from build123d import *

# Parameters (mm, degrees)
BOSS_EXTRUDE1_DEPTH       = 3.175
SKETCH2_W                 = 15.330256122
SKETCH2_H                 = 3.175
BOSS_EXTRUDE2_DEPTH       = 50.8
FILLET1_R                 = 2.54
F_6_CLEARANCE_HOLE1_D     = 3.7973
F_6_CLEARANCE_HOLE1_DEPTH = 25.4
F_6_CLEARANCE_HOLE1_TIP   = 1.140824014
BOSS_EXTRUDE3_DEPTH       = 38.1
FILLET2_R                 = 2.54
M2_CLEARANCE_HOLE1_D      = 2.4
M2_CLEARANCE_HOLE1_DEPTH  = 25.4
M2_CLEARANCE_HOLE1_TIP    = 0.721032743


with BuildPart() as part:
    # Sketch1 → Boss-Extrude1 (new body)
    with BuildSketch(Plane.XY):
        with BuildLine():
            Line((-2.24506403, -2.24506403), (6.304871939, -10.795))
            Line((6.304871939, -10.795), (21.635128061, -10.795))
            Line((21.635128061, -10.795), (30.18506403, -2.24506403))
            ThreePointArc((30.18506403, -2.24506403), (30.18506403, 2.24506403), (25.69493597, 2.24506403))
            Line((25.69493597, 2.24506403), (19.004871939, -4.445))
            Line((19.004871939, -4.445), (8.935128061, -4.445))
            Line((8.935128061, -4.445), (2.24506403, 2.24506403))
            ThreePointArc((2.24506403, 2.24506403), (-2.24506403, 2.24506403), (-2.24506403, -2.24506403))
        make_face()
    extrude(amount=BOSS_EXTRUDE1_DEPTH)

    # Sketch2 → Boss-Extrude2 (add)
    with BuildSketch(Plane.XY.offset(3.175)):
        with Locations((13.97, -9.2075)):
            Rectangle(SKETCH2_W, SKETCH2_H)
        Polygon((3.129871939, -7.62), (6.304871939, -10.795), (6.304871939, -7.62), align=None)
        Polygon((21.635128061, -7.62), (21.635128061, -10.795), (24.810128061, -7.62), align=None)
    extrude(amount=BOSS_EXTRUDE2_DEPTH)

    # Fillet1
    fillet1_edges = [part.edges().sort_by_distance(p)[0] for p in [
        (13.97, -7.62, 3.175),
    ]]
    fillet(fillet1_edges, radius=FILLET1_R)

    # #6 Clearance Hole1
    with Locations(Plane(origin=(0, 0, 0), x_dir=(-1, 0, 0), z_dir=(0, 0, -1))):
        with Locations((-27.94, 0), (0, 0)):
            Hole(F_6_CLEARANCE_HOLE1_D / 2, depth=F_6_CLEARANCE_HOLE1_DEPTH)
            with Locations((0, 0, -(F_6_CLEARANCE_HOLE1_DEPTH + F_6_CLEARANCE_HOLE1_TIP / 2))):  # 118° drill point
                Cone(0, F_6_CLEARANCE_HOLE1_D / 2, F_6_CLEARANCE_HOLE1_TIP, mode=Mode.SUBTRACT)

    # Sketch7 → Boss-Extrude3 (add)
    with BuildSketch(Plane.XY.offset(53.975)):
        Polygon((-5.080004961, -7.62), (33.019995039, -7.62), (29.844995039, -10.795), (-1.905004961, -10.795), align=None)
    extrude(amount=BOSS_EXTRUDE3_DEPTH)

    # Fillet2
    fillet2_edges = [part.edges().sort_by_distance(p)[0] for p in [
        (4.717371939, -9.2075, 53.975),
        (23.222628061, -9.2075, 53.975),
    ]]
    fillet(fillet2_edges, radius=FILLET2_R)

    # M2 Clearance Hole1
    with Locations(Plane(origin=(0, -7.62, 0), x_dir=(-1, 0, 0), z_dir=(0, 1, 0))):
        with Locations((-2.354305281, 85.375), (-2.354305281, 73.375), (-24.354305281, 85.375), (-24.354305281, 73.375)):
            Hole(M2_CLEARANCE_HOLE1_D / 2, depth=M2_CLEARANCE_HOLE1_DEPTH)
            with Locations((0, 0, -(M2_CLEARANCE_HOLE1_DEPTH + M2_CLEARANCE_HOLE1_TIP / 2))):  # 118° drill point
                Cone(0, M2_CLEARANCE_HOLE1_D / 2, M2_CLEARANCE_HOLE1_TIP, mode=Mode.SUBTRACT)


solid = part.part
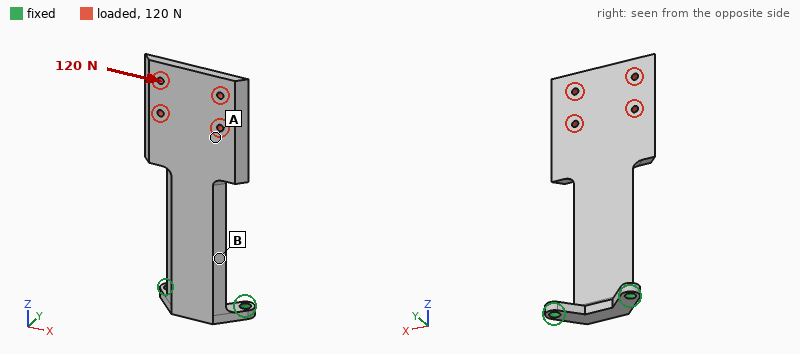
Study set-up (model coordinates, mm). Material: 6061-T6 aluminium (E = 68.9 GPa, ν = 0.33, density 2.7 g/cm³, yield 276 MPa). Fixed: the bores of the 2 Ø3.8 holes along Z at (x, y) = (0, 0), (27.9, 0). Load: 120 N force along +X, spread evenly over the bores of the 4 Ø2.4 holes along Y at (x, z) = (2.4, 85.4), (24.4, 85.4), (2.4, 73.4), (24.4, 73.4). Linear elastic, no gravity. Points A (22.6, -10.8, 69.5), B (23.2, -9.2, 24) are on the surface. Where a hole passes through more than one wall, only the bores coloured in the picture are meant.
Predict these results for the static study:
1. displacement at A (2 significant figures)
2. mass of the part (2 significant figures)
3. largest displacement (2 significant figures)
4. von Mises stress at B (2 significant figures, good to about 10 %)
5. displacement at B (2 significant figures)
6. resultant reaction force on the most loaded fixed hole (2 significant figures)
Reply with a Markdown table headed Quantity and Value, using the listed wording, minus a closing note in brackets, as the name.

| Quantity | Value |
|---|---|
| displacement at A | 0.36 mm |
| mass of the part | 21 g |
| largest displacement | 0.52 mm |
| von Mises stress at B | 35 MPa |
| displacement at B | 0.11 mm |
| resultant reaction force on the most loaded fixed hole | 400 N |
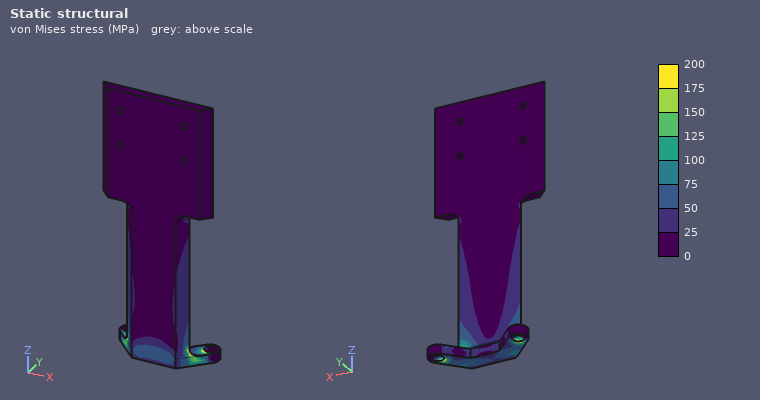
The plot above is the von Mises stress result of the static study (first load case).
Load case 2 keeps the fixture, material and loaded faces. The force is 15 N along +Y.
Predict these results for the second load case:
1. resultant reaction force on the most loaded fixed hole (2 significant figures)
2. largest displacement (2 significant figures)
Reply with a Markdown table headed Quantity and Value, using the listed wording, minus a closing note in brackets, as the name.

| Quantity | Value |
|---|---|
| resultant reaction force on the most loaded fixed hole | 17 N |
| largest displacement | 1.2 mm |
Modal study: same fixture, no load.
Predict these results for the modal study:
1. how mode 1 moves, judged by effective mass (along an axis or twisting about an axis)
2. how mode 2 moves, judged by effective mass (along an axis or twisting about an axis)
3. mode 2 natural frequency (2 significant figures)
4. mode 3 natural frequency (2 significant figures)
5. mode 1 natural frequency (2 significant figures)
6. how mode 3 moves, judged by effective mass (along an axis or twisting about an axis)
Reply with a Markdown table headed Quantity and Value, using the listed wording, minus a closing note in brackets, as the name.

| Quantity | Value |
|---|---|
| how mode 1 moves, judged by effective mass | along Y |
| how mode 2 moves, judged by effective mass | along X |
| mode 2 natural frequency | 820 Hz |
| mode 3 natural frequency | 1300 Hz |
| mode 1 natural frequency | 200 Hz |
| how mode 3 moves, judged by effective mass | twisting about Z |
